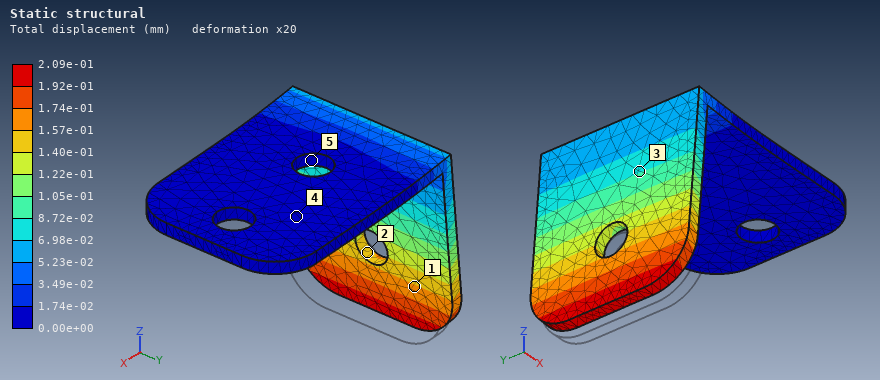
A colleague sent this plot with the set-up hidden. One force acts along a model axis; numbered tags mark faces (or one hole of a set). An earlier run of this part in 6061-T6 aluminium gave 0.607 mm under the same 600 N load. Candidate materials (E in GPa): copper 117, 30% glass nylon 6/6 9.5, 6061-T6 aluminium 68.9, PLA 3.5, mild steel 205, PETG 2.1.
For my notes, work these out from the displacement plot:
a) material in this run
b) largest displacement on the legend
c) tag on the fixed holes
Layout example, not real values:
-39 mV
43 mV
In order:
mild steel
2.09e-01 mm
5
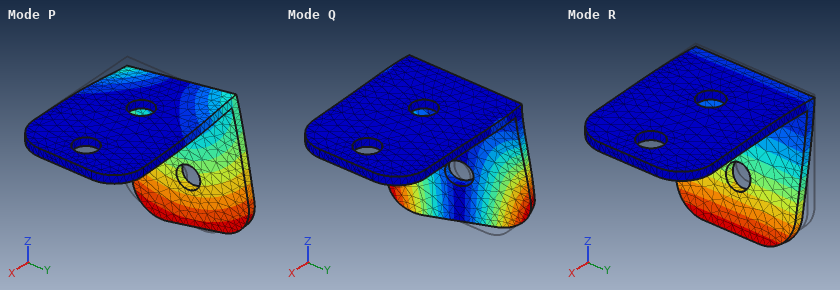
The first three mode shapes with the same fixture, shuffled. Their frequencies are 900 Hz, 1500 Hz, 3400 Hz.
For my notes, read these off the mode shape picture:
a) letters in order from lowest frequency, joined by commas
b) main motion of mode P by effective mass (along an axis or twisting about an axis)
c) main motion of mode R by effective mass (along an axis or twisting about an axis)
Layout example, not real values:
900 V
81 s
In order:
R, P, Q
along Y
along X
